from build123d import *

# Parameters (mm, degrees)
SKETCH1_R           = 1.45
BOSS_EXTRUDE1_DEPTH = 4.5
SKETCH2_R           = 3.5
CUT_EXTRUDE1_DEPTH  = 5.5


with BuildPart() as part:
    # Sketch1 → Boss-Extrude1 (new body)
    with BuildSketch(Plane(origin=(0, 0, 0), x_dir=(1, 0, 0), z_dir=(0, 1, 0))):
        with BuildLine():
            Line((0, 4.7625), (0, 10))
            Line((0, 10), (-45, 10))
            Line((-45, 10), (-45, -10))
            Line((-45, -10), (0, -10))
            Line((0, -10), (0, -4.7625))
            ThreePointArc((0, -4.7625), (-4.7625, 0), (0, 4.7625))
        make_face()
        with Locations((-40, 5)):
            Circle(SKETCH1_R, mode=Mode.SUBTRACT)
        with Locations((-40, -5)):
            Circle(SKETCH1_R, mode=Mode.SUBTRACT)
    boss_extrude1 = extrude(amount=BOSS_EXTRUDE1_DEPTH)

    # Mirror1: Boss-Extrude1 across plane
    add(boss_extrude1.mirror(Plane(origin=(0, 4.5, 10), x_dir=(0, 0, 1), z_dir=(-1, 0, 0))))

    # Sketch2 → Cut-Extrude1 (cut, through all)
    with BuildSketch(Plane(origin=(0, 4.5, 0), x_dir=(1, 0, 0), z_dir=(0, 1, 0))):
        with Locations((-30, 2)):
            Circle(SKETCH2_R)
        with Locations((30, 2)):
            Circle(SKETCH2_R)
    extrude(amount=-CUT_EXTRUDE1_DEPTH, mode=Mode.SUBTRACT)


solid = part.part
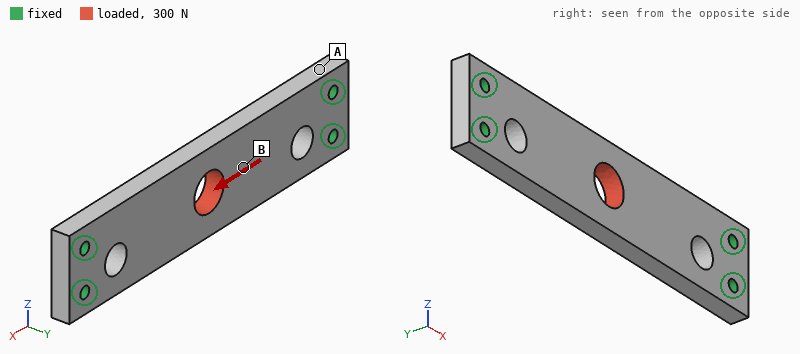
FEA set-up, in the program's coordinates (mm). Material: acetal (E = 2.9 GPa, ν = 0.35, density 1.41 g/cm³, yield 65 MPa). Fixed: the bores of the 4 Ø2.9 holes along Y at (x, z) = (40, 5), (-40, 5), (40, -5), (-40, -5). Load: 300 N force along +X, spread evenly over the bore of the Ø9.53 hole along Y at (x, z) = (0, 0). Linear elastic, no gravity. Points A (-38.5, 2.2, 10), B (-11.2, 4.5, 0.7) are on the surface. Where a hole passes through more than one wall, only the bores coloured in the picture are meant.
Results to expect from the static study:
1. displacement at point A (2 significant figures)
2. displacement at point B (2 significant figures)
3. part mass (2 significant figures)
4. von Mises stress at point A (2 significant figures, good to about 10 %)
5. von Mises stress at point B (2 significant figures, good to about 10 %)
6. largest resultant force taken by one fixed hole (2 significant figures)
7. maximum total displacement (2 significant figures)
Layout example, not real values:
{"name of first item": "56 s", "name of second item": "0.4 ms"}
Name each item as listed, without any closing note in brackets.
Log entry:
{"displacement at point A": "4.4 µm", "displacement at point B": "22 µm", "part mass": "10 g", "von Mises stress at point A": "1.1 MPa", "von Mises stress at point B": "2.0 MPa", "largest resultant force taken by one fixed hole": "84 N", "maximum total displacement": "29 µm"}
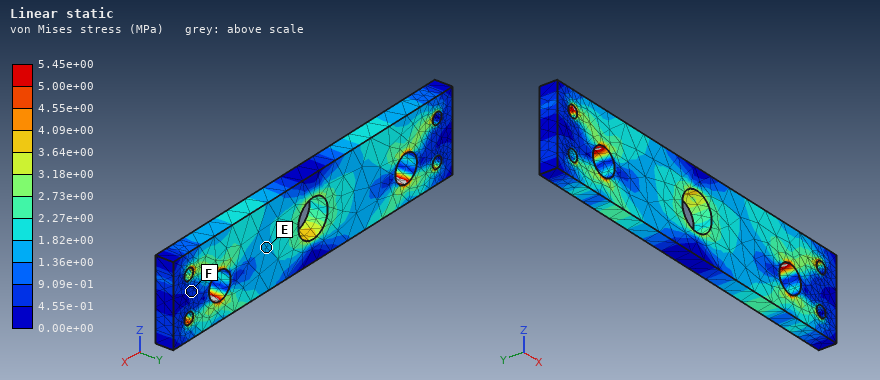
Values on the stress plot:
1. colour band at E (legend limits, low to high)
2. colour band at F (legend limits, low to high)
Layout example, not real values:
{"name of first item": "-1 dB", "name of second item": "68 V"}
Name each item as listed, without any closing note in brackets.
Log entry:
{"colour band at E": "1.36e+00 to 1.82e+00 MPa", "colour band at F": "4.55e-01 to 9.09e-01 MPa"}
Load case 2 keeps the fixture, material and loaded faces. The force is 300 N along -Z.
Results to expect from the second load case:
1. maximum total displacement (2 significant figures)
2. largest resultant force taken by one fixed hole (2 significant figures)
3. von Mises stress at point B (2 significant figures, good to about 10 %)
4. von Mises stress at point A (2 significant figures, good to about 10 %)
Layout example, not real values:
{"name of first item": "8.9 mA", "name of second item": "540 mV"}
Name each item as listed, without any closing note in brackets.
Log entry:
{"maximum total displacement": "0.21 mm", "largest resultant force taken by one fixed hole": "240 N", "von Mises stress at point B": "4.1 MPa", "von Mises stress at point A": "6.9 MPa"}
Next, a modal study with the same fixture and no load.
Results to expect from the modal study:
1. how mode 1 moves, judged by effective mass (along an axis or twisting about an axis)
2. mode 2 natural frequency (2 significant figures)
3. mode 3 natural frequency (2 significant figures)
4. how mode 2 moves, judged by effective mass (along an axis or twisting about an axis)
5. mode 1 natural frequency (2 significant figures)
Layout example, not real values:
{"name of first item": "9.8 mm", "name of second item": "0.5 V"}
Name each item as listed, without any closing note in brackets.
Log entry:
{"how mode 1 moves, judged by effective mass": "along Y", "mode 2 natural frequency": "2400 Hz", "mode 3 natural frequency": "2700 Hz", "how mode 2 moves, judged by effective mass": "twisting about X", "mode 1 natural frequency": "980 Hz"}
